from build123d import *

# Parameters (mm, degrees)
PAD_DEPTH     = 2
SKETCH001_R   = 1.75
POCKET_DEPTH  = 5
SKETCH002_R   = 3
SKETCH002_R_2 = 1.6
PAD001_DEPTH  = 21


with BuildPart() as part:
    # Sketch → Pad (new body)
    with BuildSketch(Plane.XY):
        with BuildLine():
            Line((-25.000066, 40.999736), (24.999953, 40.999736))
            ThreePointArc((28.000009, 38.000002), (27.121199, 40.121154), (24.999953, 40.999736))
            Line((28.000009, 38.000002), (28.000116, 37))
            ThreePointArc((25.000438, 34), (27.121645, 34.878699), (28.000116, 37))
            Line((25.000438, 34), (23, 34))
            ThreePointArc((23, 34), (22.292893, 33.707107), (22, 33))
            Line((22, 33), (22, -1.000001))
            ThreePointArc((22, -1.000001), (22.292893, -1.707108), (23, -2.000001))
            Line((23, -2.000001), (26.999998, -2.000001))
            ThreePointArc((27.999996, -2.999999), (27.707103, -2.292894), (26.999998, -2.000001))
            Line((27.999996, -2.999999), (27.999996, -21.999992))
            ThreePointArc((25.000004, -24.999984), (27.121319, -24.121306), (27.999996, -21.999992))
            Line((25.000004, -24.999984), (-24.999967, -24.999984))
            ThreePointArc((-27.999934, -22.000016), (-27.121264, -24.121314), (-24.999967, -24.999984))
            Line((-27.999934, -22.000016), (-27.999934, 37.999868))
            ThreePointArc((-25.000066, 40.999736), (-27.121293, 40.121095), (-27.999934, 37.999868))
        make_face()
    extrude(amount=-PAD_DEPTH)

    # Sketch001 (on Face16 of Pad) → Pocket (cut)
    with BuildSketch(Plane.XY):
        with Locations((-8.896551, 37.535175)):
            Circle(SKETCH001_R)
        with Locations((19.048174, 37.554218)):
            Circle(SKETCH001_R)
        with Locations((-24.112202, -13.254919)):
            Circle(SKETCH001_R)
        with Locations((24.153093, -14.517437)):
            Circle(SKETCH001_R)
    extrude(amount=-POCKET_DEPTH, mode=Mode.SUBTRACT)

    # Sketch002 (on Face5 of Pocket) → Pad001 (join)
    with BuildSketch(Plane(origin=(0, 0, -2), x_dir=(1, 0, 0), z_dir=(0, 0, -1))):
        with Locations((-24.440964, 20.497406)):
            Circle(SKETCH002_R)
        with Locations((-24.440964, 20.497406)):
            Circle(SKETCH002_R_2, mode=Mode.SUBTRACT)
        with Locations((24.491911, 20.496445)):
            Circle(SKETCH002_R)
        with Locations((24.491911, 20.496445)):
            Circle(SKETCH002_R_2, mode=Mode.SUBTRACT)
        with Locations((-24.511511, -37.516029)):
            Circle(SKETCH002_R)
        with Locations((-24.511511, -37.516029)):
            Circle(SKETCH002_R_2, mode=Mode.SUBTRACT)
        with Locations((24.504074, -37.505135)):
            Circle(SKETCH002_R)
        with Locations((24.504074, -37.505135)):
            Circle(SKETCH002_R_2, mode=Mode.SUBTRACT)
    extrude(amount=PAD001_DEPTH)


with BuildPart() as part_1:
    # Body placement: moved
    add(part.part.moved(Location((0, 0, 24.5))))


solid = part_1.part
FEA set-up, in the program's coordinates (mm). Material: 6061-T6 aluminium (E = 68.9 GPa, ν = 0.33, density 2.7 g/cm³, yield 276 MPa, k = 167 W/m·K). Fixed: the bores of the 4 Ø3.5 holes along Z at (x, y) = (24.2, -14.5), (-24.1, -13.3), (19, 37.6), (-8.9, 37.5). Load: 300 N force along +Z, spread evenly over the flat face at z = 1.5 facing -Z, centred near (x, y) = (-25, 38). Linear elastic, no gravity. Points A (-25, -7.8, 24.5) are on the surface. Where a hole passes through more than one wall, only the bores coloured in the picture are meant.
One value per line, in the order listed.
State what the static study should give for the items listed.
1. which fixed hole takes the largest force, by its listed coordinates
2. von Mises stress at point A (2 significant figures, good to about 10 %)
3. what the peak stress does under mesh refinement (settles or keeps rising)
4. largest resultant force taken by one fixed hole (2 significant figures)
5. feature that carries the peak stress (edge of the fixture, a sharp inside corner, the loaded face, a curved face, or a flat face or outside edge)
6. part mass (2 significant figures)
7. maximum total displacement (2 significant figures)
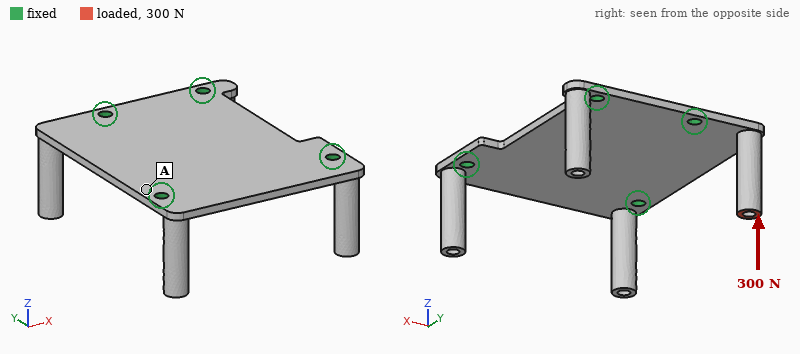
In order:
(-8.9, 37.5)
38 MPa
keeps rising
330 N
edge of the fixture
23 g
0.94 mm
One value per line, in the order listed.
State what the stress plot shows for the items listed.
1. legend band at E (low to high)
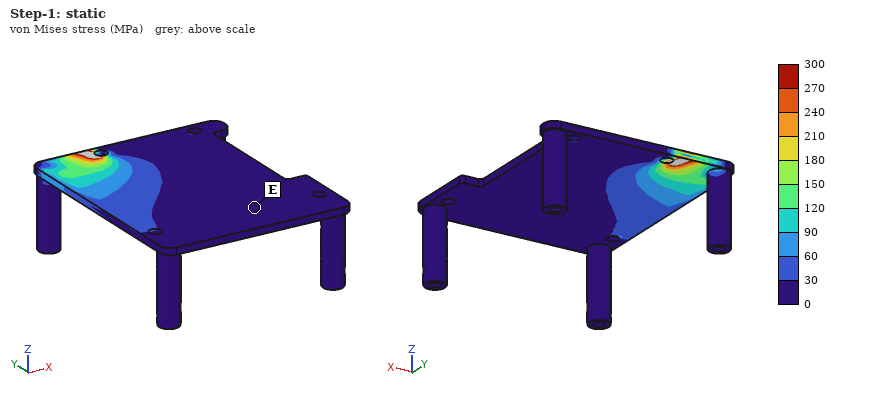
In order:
0 to 30 MPa
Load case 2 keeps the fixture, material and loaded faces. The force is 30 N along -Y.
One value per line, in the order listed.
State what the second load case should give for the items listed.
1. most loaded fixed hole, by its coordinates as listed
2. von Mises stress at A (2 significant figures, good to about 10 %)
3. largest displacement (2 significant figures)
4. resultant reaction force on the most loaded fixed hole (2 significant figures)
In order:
(-8.9, 37.5)
9.3 MPa
0.19 mm
20 N
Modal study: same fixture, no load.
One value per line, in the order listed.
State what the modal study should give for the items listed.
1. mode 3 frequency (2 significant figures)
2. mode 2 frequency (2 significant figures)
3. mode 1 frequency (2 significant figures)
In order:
3400 Hz
2800 Hz
2200 Hz
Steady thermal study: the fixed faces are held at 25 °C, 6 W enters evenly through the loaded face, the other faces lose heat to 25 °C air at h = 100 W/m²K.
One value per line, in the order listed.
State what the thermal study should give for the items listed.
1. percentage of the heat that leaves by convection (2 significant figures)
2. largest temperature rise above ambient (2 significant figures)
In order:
42 %
43 K
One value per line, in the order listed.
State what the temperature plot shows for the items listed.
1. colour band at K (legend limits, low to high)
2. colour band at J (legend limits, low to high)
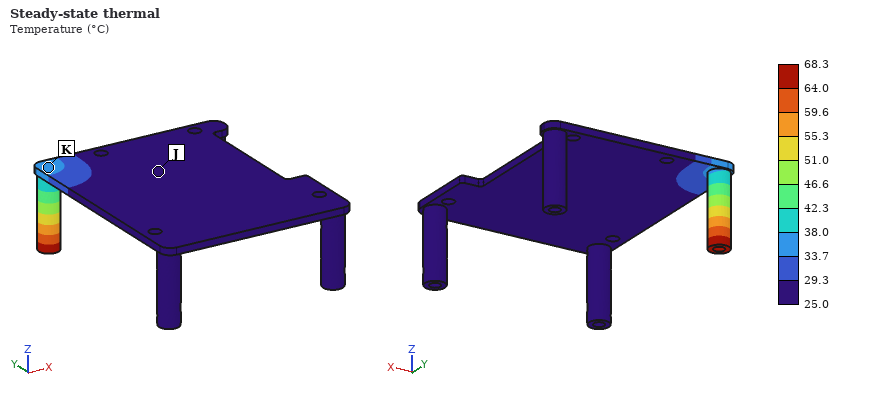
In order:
33.7 to 38.0 °C
25.0 to 29.3 °C
